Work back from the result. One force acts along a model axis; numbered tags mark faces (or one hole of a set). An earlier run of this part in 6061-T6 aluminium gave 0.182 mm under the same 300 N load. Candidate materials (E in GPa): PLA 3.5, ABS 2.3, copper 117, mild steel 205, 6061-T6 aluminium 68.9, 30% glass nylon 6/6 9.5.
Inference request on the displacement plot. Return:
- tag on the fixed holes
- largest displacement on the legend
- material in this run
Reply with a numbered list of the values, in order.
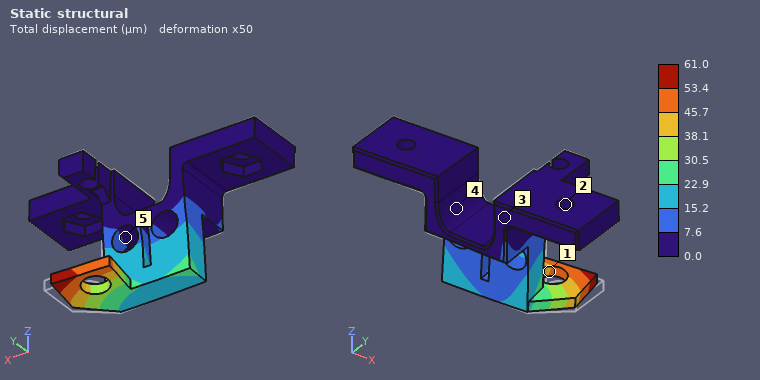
1. 2
2. 61.0 µm
3. mild steel
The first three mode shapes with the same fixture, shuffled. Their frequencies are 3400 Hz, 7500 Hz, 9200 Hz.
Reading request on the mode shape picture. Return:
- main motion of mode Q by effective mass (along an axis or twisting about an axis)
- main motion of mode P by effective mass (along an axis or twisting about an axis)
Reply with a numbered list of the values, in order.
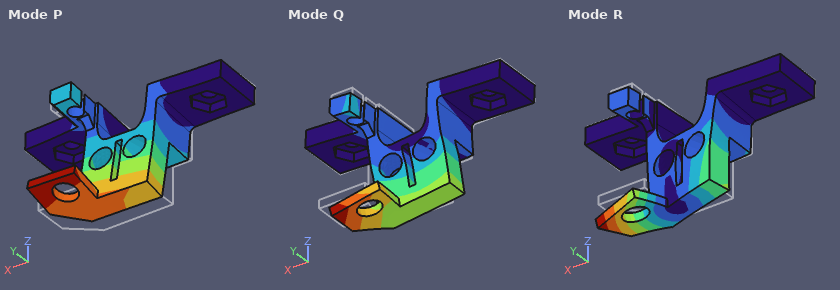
1. along X
2. along Y
